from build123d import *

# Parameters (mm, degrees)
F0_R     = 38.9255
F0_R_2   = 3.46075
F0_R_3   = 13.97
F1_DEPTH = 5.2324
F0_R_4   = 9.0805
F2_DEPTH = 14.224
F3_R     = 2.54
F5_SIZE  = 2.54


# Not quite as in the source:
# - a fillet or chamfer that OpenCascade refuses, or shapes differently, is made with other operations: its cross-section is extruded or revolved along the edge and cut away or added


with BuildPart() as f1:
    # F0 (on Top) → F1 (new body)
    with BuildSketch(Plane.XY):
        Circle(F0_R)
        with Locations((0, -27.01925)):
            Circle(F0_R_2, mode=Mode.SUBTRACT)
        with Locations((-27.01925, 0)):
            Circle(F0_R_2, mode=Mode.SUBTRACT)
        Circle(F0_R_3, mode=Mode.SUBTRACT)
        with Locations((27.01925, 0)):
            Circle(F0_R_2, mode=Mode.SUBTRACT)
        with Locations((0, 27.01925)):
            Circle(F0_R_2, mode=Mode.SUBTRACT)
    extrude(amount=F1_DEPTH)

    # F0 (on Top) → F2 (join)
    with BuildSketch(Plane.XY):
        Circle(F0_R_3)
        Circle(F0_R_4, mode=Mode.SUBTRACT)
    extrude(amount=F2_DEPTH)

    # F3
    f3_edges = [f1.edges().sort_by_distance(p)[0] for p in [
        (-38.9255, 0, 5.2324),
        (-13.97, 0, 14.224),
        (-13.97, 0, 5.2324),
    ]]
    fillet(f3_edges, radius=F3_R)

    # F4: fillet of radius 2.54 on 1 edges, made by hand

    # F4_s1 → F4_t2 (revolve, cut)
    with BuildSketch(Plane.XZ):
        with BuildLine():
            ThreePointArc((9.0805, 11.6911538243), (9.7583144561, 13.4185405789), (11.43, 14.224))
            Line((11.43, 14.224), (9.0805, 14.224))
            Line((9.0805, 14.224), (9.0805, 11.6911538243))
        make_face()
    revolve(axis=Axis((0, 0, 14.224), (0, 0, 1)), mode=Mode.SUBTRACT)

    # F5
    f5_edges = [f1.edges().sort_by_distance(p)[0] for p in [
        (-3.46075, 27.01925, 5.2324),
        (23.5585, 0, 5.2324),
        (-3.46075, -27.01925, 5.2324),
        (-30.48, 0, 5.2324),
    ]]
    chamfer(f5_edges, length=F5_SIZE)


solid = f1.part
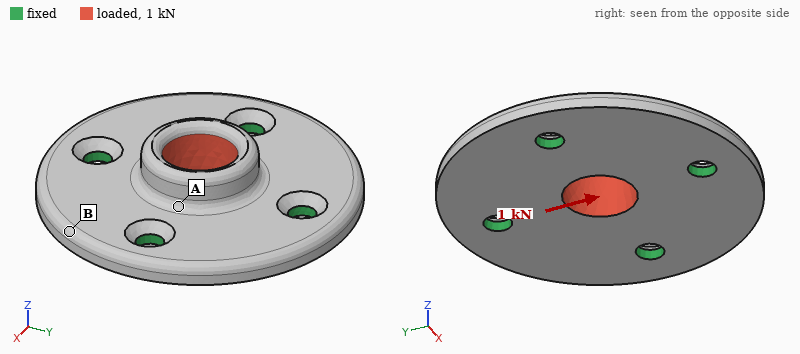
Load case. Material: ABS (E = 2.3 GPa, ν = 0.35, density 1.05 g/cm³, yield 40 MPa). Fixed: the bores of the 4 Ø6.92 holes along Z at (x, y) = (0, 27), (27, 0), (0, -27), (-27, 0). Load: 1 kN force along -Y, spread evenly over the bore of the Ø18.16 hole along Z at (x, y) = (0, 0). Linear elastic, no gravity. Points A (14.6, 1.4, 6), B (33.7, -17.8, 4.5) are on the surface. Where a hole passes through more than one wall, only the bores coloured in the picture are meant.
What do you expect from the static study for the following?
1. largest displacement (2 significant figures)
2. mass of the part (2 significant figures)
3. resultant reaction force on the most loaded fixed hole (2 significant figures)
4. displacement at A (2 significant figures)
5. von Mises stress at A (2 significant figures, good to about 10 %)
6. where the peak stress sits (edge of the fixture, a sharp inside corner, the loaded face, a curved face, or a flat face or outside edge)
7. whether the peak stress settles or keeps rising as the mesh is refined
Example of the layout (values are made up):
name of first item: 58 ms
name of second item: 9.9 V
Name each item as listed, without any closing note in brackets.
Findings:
largest displacement: 52 µm
mass of the part: 26 g
resultant reaction force on the most loaded fixed hole: 340 N
displacement at A: 27 µm
von Mises stress at A: 2.8 MPa
where the peak stress sits: edge of the fixture
whether the peak stress settles or keeps rising as the mesh is refined: keeps rising
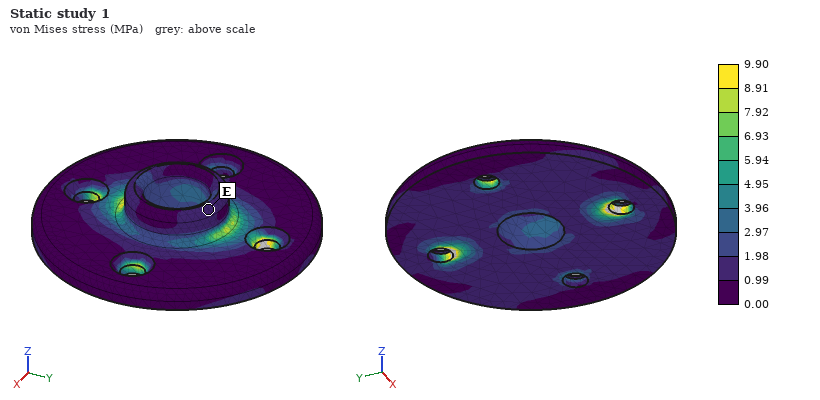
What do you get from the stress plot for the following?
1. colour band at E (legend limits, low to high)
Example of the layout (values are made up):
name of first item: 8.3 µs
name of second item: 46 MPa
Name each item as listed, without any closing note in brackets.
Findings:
colour band at E: 0.99 to 1.98 MPa
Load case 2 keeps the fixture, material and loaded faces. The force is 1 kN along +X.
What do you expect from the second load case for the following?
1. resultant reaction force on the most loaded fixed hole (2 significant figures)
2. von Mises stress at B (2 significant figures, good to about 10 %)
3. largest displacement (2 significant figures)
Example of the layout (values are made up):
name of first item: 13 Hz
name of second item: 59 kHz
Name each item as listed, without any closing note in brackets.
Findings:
resultant reaction force on the most loaded fixed hole: 340 N
von Mises stress at B: 0.84 MPa
largest displacement: 52 µm
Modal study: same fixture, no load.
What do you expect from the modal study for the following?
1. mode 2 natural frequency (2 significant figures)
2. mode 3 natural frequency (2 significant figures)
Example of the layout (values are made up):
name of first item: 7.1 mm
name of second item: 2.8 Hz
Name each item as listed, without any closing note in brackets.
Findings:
mode 2 natural frequency: 2900 Hz
mode 3 natural frequency: 2900 Hz
